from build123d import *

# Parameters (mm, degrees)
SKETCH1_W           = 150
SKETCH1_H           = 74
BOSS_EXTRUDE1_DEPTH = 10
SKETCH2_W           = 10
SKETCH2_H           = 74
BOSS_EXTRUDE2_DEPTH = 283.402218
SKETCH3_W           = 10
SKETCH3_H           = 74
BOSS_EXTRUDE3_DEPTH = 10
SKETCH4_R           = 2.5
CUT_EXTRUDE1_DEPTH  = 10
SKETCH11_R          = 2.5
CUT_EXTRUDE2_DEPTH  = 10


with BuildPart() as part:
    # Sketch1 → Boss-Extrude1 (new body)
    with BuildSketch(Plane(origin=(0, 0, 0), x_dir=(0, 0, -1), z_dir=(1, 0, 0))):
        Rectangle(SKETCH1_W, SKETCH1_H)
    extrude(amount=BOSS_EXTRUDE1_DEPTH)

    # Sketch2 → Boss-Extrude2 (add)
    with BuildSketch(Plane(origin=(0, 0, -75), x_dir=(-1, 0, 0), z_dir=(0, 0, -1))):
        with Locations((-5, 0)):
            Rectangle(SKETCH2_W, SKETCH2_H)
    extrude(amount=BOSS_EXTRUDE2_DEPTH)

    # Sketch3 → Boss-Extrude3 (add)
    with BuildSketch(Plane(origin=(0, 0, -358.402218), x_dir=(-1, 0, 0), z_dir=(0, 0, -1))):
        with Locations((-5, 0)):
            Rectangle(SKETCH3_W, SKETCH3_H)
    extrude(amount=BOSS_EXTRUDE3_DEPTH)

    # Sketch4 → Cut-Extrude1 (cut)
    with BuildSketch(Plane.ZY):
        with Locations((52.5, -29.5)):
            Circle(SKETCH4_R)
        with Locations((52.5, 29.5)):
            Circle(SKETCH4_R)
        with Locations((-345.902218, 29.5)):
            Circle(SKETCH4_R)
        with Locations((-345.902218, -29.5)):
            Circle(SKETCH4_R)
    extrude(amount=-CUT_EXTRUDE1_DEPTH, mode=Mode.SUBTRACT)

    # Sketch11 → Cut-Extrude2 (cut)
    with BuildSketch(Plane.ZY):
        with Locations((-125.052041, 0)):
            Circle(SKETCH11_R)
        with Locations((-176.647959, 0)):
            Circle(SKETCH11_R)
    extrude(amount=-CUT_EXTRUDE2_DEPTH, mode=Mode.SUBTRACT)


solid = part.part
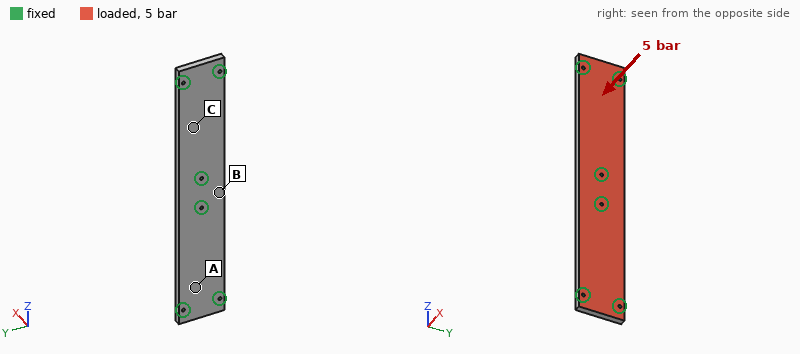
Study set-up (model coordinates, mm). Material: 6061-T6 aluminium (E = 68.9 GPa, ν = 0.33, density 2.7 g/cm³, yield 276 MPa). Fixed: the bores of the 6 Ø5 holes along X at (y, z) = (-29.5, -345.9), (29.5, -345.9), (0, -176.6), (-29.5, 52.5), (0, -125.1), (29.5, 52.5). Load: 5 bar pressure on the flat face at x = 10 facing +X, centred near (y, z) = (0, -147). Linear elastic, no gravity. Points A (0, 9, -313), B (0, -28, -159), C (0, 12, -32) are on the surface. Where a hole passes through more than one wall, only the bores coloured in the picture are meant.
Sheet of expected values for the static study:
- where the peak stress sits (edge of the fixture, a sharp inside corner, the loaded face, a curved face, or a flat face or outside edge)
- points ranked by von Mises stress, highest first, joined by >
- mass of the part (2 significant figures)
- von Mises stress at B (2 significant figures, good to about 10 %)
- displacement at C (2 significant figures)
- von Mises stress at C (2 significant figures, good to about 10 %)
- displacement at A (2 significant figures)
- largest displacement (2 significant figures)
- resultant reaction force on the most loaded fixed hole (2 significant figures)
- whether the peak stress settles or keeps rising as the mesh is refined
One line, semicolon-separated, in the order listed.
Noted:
edge of the fixture; C > B > A; 880 g; 24 MPa; 0.28 mm; 41 MPa; 0.11 mm; 0.30 mm; 4.3 kN; keeps rising
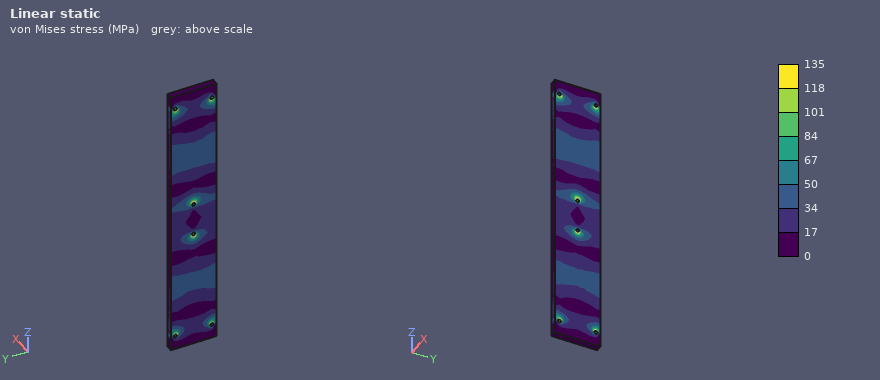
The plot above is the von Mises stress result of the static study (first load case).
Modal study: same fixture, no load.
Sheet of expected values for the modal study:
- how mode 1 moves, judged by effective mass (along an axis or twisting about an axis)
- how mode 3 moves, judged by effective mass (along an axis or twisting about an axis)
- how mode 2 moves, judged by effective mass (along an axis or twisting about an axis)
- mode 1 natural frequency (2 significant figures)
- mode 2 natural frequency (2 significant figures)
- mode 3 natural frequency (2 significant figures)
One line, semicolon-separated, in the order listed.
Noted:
along X; twisting about Z; along X; 1400 Hz; 1600 Hz; 2300 Hz
